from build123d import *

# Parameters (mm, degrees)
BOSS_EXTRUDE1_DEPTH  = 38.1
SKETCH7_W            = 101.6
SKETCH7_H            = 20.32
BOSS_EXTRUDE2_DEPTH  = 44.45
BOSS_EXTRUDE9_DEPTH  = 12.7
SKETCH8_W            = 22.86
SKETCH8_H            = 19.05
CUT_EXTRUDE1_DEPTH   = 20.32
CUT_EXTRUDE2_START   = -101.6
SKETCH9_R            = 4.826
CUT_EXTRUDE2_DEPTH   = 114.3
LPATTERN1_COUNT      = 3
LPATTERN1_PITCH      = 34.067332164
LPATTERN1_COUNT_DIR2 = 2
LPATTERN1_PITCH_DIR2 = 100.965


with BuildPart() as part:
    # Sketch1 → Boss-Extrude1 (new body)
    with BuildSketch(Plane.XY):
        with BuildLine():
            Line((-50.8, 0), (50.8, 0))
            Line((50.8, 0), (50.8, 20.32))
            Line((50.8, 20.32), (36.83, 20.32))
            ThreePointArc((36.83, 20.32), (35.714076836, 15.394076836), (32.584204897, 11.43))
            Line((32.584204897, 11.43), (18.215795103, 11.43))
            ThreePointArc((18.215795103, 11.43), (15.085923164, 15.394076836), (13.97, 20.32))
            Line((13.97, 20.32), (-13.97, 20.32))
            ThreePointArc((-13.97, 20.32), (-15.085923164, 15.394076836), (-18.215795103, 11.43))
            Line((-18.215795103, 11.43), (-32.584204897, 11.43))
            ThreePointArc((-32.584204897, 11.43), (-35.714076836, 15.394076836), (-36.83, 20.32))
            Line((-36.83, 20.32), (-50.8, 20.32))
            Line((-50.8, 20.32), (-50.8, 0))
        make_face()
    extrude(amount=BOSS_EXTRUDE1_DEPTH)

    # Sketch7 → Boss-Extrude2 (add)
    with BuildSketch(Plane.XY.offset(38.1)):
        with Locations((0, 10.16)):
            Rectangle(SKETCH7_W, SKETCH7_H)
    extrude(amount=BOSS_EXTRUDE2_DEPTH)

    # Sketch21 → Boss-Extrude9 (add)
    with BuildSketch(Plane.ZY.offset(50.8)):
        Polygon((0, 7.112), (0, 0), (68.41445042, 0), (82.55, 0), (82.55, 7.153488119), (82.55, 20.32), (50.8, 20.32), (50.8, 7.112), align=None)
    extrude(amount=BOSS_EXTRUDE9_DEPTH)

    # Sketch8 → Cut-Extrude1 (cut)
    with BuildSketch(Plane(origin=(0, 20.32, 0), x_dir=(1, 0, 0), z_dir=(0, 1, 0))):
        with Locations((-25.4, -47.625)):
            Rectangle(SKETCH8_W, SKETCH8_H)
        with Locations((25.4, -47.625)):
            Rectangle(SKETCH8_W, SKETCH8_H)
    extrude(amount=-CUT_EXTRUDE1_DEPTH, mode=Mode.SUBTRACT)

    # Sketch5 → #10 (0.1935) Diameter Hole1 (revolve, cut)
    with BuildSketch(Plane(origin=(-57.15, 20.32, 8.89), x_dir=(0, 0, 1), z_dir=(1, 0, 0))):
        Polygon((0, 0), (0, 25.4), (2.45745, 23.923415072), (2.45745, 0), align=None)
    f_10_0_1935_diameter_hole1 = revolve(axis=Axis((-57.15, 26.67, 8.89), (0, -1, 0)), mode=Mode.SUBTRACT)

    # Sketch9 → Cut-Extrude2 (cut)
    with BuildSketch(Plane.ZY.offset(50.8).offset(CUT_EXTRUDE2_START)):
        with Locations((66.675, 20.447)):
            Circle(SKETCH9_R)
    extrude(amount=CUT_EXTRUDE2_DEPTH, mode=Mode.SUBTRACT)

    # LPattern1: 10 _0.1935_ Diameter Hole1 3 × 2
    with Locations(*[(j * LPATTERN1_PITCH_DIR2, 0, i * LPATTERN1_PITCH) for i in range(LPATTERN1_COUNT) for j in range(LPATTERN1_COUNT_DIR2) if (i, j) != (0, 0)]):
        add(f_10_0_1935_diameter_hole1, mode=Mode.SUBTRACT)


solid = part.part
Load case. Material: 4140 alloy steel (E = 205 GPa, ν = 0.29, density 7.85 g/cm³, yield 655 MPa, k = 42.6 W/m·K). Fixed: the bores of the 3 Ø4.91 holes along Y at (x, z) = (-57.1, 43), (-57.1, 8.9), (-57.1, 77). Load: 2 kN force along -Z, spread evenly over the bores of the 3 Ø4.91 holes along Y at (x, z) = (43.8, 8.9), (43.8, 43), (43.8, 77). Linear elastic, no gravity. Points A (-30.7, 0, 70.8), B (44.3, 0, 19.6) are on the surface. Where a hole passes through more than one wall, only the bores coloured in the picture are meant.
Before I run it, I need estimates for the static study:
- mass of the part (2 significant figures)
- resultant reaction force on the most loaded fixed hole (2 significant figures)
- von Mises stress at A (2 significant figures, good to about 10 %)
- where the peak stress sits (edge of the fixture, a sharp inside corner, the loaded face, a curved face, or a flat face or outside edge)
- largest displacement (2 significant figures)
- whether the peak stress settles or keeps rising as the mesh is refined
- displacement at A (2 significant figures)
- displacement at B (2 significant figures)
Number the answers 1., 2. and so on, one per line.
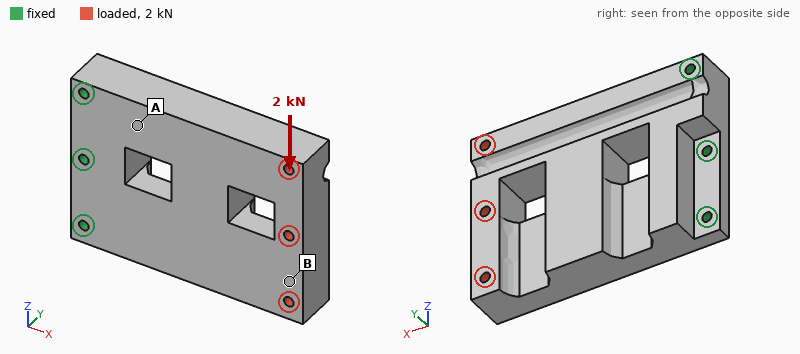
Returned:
1. 1.1 kg
2. 3.0 kN
3. 12 MPa
4. edge of the fixture
5. 23 µm
6. keeps rising
7. 3.6 µm
8. 20 µm
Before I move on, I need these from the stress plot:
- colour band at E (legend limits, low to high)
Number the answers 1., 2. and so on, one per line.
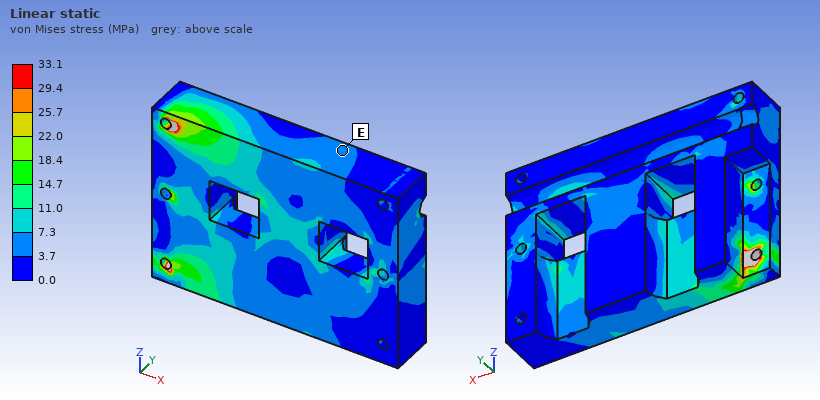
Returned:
1. 3.7 to 7.3 MPa
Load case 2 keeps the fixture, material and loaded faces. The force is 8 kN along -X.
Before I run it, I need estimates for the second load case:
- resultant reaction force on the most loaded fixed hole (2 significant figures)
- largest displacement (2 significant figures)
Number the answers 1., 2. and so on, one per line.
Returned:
1. 3.3 kN
2. 48 µm
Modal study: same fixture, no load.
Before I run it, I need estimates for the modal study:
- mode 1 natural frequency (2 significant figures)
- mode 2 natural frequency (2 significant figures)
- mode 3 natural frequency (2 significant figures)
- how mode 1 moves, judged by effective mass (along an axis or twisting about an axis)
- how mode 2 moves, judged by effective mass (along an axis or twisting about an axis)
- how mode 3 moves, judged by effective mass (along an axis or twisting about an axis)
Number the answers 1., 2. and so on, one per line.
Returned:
1. 820 Hz
2. 2700 Hz
3. 3300 Hz
4. along Y
5. twisting about X
6. along Z
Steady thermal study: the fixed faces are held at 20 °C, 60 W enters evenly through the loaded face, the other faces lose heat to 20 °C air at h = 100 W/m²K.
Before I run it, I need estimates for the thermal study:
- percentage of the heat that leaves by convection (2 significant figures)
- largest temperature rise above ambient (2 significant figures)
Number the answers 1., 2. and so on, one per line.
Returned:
1. 86 %
2. 51 K
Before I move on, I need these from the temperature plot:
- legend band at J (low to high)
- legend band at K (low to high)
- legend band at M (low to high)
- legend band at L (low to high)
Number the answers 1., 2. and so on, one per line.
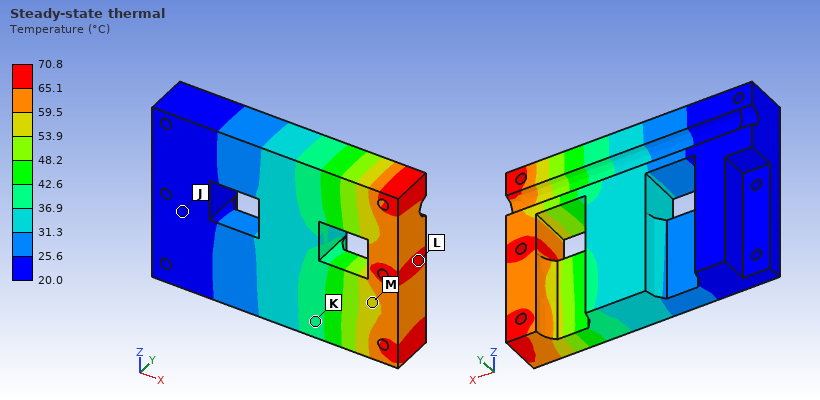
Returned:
1. 20.0 to 25.6 °C
2. 36.9 to 42.6 °C
3. 53.9 to 59.5 °C
4. 65.1 to 70.8 °C
